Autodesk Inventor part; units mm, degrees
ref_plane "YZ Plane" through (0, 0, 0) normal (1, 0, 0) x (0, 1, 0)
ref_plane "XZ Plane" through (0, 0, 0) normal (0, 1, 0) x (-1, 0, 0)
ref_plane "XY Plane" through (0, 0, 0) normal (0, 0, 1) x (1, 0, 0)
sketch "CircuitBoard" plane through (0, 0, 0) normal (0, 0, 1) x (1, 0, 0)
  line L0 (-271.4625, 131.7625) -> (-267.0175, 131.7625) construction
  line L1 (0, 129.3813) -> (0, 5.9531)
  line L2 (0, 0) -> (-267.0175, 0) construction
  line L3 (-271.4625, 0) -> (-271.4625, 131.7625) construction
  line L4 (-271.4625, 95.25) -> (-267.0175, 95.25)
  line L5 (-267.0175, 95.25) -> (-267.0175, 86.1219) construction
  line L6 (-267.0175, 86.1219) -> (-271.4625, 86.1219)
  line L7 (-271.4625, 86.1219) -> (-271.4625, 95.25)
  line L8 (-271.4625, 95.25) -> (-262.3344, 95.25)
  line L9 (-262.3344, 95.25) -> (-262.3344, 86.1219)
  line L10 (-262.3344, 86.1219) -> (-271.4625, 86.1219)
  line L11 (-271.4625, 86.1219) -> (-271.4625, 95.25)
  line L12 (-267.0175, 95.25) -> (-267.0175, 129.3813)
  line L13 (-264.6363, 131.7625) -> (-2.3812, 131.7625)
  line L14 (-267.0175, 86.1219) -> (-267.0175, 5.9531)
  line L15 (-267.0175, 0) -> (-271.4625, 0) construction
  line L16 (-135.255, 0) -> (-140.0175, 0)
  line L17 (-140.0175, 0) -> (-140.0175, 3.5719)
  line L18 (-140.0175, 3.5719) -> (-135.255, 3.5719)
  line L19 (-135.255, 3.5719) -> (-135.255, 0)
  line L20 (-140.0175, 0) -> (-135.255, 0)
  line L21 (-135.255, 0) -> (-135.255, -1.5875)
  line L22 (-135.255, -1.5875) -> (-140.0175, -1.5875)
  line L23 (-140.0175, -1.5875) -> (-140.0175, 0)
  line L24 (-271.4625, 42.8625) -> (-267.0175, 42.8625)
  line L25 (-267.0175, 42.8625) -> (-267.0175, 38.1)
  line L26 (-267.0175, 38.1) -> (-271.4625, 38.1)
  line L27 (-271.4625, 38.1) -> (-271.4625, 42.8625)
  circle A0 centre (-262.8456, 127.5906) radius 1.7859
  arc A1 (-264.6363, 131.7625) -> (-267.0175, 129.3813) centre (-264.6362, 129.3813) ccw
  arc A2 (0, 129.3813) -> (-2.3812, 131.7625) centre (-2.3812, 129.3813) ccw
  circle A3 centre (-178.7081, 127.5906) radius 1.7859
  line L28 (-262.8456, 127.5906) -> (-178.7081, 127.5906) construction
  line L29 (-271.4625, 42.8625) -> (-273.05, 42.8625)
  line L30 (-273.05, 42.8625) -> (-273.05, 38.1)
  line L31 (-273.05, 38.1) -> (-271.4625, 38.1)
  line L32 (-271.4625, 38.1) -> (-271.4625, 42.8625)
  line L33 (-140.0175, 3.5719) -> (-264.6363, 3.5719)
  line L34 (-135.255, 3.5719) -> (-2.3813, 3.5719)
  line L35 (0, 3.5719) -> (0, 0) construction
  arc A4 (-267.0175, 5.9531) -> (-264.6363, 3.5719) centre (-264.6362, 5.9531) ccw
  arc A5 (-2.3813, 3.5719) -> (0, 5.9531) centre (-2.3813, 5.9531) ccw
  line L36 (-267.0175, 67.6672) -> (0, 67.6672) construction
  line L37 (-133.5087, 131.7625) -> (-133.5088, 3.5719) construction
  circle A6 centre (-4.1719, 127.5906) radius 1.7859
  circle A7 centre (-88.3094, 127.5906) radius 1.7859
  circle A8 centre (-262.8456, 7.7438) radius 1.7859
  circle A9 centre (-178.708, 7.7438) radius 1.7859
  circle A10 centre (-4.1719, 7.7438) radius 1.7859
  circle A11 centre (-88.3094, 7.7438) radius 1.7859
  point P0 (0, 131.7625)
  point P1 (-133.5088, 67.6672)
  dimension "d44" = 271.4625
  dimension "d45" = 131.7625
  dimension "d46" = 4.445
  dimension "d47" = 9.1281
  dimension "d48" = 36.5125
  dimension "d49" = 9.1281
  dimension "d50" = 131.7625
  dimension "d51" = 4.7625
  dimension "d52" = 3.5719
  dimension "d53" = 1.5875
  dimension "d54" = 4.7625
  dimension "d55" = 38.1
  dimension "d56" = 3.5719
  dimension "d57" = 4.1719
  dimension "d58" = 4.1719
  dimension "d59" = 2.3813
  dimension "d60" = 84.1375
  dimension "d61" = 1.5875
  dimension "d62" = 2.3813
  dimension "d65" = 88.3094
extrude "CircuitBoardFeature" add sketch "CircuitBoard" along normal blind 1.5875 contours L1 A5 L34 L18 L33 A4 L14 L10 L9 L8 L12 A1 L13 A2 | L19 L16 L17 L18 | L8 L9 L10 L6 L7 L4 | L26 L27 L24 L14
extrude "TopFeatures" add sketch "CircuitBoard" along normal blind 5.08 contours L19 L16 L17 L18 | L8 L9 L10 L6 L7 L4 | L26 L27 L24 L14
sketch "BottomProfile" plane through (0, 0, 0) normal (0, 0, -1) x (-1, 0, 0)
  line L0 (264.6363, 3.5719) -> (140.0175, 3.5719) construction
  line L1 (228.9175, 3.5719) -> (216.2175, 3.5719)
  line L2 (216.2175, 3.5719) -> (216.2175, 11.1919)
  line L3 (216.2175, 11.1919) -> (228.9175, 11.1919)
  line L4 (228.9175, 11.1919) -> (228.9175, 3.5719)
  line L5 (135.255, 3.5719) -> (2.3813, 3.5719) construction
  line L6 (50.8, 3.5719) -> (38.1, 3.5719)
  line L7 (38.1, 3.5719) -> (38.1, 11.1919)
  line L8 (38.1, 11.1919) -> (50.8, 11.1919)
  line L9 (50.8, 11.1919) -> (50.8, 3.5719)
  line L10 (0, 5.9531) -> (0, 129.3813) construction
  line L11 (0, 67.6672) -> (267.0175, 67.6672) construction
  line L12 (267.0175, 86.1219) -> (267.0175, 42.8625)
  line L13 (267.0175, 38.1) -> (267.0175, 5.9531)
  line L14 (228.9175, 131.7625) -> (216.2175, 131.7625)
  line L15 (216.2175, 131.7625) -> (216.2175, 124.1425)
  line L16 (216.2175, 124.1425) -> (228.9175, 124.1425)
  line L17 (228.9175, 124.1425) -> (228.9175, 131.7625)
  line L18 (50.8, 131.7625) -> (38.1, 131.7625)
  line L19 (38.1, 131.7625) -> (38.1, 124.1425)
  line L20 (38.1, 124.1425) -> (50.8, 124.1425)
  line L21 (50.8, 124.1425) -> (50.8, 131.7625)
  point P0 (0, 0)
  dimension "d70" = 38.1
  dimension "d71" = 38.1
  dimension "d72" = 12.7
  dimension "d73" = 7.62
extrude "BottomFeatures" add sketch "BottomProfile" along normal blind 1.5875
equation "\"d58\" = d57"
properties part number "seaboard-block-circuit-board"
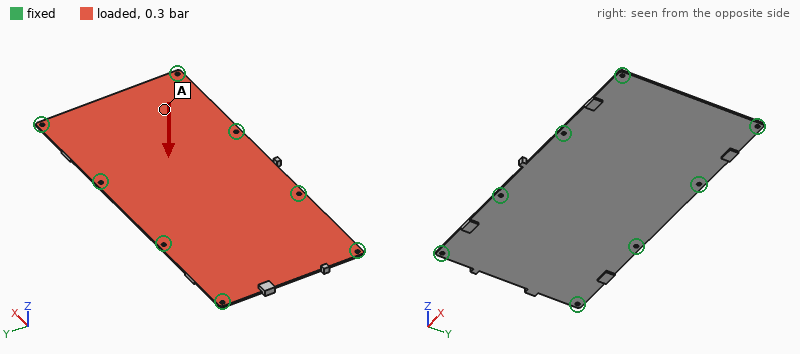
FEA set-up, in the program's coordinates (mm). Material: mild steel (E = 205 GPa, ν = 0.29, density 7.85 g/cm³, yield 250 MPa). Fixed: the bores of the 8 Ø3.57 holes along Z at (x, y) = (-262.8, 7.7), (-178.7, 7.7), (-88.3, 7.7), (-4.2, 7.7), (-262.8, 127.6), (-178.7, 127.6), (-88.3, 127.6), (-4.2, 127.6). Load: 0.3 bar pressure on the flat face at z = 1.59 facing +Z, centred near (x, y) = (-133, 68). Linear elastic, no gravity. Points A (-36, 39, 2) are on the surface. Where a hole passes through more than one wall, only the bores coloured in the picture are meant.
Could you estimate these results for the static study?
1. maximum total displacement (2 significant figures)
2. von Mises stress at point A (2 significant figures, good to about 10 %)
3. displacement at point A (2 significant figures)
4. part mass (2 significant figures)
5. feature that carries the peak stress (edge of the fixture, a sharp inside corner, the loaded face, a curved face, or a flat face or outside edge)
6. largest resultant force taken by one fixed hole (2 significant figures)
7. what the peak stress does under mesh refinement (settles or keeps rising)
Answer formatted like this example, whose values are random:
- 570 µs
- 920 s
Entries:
- 0.45 mm
- 30 MPa
- 0.31 mm
- 430 g
- edge of the fixture
- 170 N
- keeps rising
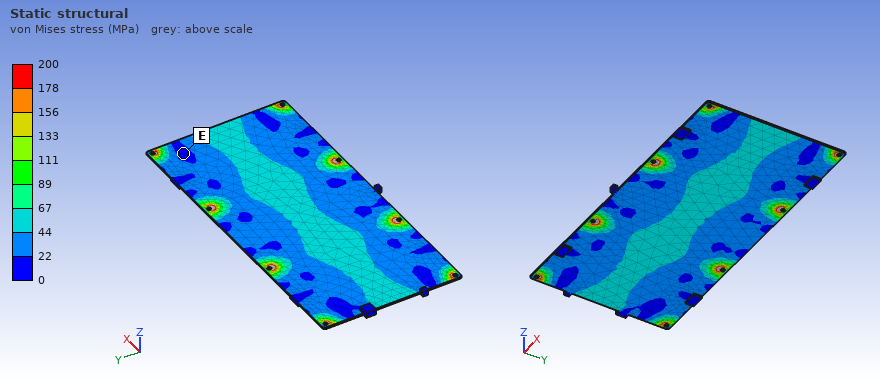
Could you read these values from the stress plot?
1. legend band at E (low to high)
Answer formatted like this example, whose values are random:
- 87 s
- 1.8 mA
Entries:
- 0 to 22 MPa
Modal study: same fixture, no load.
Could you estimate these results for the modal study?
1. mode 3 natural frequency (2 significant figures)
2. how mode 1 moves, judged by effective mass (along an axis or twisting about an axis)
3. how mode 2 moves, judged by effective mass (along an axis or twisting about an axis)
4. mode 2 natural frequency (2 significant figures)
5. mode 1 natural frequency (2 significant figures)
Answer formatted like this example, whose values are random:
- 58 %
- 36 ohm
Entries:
- 550 Hz
- along Z
- twisting about Y
- 470 Hz
- 430 Hz
